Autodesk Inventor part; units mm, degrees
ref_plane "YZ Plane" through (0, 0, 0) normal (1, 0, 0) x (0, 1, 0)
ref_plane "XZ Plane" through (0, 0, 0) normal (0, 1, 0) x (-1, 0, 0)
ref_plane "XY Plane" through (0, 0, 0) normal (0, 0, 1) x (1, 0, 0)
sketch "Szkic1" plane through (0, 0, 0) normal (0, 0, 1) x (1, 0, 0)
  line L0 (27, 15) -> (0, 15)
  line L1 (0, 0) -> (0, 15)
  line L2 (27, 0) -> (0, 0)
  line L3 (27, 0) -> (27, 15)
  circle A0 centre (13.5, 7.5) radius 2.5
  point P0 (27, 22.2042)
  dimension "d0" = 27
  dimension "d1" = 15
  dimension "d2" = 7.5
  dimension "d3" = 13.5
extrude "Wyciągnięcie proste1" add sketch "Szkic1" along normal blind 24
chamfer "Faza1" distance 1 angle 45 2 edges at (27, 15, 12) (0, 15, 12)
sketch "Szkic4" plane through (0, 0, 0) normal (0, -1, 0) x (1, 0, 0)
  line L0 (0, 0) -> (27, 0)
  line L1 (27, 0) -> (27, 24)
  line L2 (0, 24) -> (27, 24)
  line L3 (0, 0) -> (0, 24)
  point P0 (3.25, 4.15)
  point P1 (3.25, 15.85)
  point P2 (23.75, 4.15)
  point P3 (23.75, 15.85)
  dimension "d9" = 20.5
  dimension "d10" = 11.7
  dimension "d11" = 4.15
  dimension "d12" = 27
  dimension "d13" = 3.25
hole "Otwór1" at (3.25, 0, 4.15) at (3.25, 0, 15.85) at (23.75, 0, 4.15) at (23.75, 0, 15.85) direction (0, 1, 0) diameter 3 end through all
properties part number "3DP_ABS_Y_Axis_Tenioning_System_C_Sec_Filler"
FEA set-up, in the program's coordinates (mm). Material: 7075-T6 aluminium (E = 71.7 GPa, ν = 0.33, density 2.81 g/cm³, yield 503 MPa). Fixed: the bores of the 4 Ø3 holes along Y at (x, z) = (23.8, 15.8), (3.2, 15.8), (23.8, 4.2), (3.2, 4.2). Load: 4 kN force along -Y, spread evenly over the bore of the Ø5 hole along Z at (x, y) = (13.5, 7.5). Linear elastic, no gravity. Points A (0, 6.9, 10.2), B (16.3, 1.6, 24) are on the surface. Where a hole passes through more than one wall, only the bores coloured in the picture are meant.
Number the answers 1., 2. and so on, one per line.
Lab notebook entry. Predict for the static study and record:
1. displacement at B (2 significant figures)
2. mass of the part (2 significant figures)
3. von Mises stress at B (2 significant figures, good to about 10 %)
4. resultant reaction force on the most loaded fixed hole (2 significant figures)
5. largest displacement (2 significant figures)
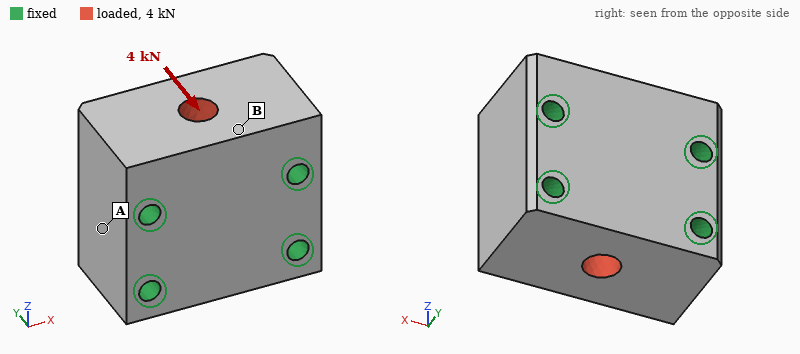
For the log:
1. 2.8 µm
2. 25 g
3. 9.6 MPa
4. 1.2 kN
5. 3.4 µm
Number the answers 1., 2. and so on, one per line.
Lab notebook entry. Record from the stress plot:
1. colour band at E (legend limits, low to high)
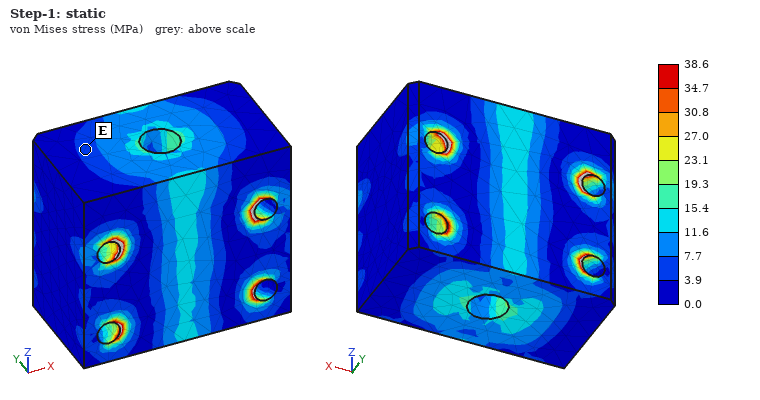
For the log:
1. 3.9 to 7.7 MPa
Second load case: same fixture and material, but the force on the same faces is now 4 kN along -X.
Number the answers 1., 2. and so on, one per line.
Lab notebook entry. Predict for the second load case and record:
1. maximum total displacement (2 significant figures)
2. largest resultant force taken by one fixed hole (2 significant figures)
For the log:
1. 1.6 µm
2. 1.2 kN
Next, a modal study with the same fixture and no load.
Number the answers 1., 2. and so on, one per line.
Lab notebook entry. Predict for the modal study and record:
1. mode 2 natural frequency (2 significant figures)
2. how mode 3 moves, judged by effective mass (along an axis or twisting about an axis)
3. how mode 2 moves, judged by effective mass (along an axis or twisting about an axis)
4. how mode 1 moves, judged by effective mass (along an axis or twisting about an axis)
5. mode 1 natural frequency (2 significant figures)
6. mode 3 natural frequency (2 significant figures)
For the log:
1. 69 kHz
2. along Y
3. along Z
4. along Y
5. 59 kHz
6. 72 kHz
